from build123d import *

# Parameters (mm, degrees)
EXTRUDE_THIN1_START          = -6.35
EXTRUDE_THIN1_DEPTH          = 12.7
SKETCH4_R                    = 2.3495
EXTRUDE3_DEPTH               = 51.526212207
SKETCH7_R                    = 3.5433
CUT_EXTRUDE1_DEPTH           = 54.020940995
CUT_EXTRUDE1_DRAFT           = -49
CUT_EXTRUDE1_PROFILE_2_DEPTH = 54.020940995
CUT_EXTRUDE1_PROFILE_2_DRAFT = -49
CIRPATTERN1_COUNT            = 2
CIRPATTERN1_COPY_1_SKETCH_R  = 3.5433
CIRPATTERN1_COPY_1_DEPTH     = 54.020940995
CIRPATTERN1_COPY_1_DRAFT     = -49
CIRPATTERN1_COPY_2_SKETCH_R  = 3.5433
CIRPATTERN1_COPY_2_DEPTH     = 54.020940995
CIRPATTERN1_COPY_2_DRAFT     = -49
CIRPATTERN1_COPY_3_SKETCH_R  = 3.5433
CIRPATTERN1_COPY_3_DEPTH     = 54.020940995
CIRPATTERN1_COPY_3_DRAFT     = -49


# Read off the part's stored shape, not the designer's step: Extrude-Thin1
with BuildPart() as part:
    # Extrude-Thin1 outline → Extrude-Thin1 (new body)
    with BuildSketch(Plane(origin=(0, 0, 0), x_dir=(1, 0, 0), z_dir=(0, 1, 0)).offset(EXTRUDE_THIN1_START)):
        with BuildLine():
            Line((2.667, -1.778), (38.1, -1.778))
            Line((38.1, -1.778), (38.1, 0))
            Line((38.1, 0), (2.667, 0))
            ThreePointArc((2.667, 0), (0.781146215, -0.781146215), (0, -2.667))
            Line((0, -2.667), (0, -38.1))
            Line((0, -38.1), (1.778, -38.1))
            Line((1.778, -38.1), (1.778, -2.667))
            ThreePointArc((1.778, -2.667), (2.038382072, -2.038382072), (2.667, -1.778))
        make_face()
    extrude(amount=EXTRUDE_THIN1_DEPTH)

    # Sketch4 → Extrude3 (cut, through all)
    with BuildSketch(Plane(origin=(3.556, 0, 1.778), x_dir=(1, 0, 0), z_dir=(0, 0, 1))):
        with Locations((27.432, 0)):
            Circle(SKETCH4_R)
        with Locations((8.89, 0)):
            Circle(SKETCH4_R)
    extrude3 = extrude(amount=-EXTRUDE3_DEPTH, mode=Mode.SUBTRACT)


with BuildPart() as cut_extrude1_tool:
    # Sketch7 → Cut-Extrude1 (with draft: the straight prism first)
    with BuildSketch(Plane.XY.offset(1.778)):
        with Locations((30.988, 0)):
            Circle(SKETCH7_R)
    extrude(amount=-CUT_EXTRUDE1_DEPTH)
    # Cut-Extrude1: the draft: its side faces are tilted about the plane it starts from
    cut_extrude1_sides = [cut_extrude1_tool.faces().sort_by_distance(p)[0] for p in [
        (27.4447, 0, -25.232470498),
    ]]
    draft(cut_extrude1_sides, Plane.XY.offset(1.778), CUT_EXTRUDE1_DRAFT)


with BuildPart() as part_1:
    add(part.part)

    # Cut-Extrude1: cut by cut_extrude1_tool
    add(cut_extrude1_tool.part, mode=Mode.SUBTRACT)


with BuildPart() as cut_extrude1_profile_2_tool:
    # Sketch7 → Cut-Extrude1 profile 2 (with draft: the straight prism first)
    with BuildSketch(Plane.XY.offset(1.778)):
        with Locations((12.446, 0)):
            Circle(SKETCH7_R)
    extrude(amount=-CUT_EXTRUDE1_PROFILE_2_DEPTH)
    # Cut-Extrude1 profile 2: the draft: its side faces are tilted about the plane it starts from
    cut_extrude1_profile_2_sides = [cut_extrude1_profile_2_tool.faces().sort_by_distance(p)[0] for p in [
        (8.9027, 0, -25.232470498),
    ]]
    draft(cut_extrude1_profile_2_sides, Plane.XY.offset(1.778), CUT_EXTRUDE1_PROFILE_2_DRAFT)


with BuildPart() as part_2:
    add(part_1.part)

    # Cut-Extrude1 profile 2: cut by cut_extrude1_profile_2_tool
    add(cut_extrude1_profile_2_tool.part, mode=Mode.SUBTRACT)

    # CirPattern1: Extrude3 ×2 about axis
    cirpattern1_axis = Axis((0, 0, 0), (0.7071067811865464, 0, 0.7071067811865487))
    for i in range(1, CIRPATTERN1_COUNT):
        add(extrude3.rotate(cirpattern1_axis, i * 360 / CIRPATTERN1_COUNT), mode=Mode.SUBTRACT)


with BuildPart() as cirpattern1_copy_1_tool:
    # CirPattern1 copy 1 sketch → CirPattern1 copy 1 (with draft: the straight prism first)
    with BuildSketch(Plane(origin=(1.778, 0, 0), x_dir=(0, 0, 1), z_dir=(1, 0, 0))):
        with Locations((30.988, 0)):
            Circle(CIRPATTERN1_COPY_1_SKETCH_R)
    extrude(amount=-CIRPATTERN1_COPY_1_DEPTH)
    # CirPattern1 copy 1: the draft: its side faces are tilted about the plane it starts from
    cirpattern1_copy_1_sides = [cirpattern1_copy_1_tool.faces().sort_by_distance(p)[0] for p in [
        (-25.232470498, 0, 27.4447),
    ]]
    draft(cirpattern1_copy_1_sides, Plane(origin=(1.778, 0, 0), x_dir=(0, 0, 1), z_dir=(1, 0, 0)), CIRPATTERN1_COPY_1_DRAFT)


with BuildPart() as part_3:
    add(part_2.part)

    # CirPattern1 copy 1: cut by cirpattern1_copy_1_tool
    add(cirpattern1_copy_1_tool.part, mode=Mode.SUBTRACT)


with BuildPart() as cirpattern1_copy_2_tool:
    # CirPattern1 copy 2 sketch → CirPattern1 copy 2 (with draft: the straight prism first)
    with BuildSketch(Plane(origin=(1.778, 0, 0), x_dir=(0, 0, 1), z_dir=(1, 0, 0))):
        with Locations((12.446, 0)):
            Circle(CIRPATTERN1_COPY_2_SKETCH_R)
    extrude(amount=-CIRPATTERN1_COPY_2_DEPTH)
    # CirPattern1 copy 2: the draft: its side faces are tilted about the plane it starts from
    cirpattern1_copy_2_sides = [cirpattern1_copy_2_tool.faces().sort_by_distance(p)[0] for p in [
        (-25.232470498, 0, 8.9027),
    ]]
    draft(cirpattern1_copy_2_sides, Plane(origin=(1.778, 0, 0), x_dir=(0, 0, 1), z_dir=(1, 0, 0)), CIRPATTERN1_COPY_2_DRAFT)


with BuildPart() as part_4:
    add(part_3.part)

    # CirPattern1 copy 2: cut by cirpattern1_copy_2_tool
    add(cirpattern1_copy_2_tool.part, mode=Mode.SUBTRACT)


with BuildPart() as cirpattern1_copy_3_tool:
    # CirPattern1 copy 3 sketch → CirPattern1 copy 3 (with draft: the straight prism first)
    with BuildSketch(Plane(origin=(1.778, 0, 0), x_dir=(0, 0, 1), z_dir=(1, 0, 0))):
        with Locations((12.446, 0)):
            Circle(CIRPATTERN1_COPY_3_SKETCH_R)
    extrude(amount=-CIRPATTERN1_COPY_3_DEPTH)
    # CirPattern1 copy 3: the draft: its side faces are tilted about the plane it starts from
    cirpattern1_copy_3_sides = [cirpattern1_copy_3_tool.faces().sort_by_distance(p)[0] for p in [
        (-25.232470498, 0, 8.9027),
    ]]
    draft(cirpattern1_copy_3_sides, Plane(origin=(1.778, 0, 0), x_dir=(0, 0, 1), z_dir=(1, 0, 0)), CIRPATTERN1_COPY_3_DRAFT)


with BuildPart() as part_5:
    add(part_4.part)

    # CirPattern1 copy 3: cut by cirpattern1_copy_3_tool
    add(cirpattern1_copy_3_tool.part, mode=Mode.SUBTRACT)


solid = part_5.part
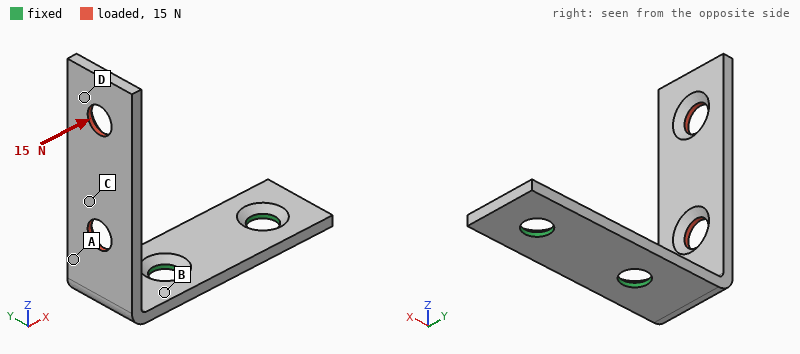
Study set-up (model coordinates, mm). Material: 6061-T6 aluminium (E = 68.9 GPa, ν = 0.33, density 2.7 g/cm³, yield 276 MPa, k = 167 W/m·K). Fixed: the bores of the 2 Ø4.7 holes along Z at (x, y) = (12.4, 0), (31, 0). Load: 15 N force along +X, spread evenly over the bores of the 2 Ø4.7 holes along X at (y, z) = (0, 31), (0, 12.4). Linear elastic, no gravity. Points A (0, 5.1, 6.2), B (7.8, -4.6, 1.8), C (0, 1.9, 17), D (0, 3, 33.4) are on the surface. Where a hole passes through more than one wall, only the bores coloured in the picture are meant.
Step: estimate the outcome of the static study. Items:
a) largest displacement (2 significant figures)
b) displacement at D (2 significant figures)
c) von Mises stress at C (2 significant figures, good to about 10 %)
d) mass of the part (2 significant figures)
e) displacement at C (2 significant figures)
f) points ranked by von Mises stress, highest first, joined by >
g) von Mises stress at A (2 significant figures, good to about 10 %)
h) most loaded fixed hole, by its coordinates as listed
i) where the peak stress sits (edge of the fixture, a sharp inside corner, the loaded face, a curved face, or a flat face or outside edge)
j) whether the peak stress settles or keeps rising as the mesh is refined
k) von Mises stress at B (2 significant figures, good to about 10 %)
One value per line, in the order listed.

0.62 mm
0.53 mm
15 MPa
4.0 g
0.23 mm
B > A > C > D
37 MPa
(31, 0)
edge of the fixture
keeps rising
51 MPa
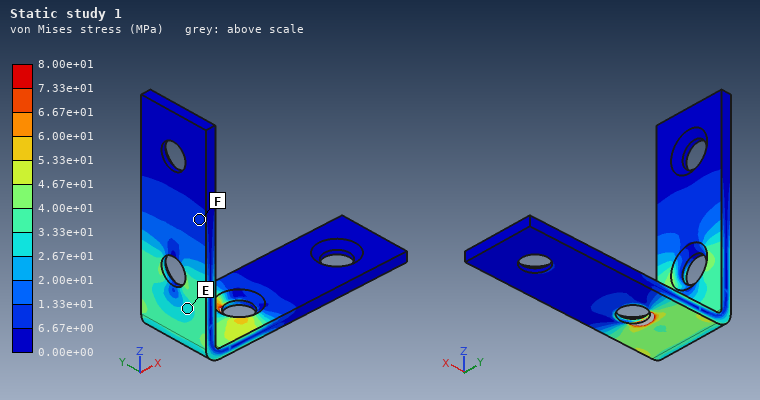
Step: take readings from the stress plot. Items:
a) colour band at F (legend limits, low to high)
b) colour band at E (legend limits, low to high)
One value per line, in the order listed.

6.67e+00 to 1.33e+01 MPa
2.67e+01 to 3.33e+01 MPa
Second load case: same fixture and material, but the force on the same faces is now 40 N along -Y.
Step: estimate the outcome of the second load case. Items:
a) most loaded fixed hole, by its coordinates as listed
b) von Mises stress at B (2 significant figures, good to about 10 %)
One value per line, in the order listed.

(12.4, 0)
71 MPa
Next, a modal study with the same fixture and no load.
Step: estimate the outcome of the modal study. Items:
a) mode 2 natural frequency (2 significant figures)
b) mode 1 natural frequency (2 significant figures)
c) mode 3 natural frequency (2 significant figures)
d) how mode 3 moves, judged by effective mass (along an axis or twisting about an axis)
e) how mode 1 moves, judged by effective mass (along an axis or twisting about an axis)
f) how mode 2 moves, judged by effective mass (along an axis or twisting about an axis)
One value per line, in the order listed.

1200 Hz
720 Hz
3500 Hz
along Z
along X
along Y
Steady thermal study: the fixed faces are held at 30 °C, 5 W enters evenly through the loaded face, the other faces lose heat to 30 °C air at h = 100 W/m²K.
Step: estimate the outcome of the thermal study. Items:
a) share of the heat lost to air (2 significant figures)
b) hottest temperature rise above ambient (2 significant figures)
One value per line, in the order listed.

45 %
28 K
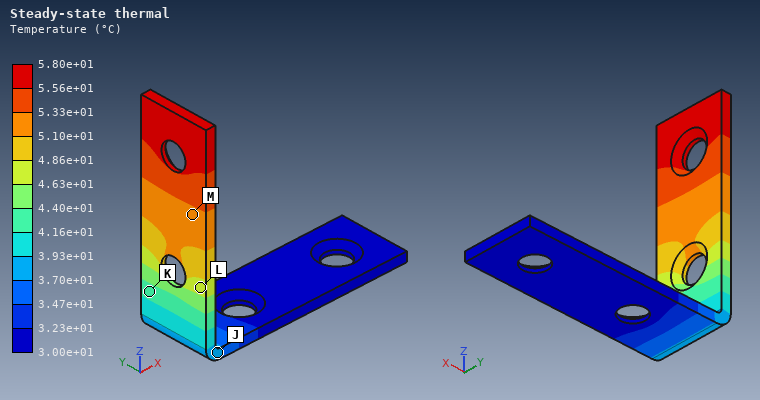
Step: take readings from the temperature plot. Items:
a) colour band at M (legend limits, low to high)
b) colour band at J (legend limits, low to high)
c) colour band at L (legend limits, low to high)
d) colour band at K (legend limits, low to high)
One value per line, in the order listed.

5.10e+01 to 5.33e+01 °C
3.70e+01 to 3.93e+01 °C
4.63e+01 to 4.86e+01 °C
4.16e+01 to 4.40e+01 °C
